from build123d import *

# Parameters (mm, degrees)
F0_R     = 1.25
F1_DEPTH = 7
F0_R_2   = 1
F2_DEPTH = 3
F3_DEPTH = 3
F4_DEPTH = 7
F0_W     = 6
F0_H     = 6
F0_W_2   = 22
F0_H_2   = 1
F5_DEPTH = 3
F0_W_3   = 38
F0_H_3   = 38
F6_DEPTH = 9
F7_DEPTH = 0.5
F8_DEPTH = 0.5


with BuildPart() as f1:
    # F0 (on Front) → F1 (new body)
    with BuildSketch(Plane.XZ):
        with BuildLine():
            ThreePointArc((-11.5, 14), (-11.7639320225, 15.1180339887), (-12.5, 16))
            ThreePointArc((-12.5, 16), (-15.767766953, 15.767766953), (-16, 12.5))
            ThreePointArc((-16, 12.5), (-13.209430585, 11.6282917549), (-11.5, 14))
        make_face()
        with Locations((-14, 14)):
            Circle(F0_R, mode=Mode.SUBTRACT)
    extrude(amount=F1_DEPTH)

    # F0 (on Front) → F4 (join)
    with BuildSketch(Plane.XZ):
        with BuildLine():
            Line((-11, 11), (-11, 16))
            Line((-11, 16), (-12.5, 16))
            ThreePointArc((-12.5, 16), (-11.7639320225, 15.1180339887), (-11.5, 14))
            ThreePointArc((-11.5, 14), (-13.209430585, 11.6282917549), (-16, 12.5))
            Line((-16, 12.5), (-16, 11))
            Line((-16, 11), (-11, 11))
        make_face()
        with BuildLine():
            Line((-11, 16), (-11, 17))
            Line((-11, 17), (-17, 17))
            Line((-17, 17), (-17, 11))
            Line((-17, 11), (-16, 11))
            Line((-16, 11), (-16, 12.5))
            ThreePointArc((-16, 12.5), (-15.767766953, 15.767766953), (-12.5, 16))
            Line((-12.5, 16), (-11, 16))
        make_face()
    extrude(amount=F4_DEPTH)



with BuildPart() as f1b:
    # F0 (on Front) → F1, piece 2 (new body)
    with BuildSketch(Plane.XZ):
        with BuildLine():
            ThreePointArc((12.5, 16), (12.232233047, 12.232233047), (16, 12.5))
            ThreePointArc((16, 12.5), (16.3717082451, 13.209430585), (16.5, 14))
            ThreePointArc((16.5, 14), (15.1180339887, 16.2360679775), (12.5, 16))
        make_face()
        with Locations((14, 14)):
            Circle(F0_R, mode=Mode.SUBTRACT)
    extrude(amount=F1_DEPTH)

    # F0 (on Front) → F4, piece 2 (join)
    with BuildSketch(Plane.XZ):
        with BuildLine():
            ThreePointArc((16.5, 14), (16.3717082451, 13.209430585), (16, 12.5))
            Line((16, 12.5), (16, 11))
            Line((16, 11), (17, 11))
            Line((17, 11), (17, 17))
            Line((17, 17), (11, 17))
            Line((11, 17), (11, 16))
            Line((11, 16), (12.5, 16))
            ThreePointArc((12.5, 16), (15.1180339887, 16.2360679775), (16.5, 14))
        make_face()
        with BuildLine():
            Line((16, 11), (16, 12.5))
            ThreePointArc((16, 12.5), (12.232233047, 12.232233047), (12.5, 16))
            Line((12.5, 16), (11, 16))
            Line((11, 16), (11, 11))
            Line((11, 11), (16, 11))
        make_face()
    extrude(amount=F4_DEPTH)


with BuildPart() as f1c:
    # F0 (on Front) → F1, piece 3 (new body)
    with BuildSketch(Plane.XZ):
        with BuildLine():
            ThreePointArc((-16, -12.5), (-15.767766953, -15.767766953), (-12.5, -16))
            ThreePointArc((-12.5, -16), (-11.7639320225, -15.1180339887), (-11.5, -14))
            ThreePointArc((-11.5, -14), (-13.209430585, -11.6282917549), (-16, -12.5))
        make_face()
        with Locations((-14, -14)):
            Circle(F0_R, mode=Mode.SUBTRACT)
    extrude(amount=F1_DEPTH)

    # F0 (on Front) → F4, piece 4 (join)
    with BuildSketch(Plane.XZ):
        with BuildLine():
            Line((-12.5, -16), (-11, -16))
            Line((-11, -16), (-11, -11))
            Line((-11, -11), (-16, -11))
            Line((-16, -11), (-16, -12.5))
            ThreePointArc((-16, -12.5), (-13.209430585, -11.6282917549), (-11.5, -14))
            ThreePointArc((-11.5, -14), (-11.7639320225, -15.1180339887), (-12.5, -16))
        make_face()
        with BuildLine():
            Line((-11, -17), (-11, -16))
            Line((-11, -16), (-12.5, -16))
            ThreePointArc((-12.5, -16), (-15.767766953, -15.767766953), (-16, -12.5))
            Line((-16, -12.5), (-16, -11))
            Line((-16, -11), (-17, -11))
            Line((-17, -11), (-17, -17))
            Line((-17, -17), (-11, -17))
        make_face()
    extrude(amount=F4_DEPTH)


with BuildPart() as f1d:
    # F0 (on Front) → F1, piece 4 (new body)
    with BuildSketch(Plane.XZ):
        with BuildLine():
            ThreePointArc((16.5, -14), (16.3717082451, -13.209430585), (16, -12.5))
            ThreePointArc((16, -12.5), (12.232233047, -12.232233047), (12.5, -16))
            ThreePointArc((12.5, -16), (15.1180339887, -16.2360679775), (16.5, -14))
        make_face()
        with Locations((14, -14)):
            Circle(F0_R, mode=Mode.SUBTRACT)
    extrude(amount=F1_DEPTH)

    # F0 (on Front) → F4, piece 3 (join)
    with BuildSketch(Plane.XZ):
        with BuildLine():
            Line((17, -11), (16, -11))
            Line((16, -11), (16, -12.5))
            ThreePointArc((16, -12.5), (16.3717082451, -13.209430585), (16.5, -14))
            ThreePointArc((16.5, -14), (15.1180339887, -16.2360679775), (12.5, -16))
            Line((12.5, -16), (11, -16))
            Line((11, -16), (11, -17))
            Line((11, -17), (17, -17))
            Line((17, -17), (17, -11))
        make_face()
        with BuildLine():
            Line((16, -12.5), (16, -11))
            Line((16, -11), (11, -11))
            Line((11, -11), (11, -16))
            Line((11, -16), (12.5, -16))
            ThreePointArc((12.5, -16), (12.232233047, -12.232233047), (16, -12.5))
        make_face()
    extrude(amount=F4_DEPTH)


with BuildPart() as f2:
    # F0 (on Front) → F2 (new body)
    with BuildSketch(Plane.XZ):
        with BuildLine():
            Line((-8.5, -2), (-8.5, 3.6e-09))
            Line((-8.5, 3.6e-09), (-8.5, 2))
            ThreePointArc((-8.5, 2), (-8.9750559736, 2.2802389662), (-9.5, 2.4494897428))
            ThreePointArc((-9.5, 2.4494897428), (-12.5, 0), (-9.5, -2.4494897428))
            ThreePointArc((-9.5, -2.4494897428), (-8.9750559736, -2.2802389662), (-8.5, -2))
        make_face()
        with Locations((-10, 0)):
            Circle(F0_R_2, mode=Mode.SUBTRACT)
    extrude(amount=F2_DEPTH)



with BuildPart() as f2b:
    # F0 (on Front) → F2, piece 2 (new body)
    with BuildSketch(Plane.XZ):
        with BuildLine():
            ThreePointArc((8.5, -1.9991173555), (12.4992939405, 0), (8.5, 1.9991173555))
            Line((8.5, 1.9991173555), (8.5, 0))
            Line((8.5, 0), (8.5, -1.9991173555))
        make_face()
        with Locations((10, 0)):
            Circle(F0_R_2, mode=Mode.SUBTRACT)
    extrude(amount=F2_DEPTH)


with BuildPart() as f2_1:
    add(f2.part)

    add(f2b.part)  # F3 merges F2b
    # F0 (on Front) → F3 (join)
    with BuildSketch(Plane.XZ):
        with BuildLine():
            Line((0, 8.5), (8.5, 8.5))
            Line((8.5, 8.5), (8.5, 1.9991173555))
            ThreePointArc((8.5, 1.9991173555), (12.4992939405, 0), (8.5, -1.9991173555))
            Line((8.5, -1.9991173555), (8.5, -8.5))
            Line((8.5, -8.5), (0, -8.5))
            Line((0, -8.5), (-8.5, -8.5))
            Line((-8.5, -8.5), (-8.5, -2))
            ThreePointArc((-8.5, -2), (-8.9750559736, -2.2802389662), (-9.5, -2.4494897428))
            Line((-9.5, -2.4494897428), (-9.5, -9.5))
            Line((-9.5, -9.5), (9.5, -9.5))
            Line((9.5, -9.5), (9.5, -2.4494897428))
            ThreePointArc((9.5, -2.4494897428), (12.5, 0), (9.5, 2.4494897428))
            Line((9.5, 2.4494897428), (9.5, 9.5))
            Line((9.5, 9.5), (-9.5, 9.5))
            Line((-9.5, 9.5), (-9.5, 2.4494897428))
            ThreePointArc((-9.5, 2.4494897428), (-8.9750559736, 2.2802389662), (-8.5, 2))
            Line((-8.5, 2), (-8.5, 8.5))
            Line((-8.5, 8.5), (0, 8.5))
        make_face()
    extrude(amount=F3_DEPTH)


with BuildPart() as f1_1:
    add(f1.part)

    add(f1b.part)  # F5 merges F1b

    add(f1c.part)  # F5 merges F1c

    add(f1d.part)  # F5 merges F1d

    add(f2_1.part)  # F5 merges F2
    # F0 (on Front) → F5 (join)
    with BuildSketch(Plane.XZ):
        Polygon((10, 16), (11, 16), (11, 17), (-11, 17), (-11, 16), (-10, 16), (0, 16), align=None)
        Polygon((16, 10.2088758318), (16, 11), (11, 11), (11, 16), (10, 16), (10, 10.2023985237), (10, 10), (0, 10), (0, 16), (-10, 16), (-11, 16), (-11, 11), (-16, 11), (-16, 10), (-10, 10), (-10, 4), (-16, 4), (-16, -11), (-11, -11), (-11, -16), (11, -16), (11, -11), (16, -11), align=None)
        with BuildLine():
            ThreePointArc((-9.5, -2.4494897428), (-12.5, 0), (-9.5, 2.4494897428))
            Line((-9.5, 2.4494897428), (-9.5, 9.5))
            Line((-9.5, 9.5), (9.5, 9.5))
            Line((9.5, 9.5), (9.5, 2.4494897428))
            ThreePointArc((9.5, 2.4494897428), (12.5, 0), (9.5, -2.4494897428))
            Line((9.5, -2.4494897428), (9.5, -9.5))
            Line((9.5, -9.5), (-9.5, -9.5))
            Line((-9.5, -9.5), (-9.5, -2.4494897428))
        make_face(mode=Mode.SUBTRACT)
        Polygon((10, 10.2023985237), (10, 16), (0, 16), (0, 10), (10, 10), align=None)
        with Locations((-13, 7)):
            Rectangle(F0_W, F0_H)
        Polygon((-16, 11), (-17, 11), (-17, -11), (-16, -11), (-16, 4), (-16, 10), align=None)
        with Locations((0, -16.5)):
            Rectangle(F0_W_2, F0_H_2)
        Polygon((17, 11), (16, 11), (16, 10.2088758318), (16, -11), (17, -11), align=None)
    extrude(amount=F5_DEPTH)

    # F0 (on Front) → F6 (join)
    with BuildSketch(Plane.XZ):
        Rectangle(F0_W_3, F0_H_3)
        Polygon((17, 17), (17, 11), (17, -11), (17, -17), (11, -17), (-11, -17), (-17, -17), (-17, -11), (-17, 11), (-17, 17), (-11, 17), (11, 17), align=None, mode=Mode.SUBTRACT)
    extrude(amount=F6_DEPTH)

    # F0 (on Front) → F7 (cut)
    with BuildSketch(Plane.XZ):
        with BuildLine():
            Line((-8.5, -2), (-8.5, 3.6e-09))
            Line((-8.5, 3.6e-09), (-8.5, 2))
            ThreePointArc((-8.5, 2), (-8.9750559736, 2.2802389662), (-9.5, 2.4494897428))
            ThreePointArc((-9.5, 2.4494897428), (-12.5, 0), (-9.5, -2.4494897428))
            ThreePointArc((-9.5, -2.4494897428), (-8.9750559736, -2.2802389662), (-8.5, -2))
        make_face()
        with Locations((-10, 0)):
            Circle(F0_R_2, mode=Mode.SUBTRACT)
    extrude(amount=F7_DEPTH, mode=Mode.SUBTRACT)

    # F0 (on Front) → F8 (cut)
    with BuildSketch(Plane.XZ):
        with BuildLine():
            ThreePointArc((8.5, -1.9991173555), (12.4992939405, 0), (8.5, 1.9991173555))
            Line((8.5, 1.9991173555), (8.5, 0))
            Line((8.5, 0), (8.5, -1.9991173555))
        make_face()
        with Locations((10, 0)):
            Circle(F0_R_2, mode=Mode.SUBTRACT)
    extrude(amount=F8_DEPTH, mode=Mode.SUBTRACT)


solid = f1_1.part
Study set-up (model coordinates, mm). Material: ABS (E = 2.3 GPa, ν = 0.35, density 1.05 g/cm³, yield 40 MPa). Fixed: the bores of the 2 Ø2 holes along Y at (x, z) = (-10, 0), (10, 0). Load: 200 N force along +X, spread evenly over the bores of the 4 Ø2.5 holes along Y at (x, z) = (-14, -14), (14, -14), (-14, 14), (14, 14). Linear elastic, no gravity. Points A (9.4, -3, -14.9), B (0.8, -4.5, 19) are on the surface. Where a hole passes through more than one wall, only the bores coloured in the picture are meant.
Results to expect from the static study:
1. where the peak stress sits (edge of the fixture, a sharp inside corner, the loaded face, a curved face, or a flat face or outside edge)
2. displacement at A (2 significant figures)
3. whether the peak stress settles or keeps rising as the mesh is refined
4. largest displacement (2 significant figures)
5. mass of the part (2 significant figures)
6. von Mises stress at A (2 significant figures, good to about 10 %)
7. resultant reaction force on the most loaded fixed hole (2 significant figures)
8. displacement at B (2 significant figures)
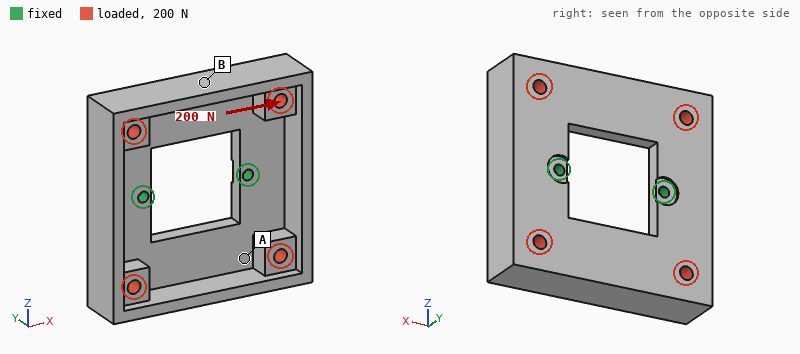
edge of the fixture
0.061 mm
keeps rising
0.12 mm
5.9 g
2.0 MPa
100 N
0.059 mm
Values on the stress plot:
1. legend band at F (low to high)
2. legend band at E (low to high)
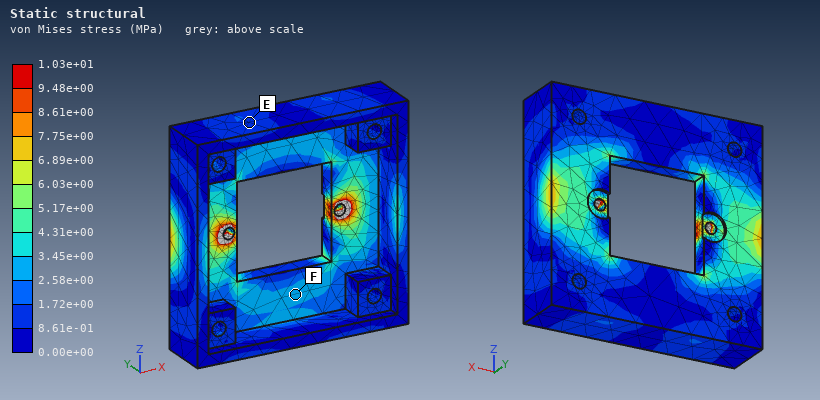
2.58e+00 to 3.45e+00 MPa
8.61e-01 to 1.72e+00 MPa
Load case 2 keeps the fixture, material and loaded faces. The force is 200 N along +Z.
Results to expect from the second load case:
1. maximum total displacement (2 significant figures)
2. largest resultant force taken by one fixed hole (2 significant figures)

0.35 mm
100 N
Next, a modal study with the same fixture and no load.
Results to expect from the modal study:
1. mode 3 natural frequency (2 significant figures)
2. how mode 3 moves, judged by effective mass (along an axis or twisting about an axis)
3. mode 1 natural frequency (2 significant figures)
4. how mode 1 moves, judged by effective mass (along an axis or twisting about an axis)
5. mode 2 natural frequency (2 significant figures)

2000 Hz
along Y
770 Hz
twisting about X
1600 Hz
